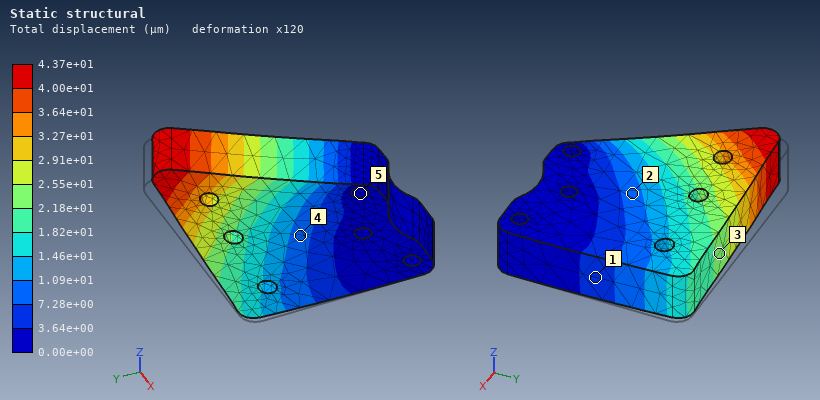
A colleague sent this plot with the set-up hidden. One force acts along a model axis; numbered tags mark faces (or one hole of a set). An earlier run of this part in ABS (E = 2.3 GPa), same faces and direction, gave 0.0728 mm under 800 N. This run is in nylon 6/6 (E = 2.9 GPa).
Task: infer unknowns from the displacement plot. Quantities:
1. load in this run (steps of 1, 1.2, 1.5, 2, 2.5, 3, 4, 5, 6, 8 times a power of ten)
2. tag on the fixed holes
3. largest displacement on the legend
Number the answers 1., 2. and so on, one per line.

1. 600 N
2. 5
3. 4.37e+01 µm
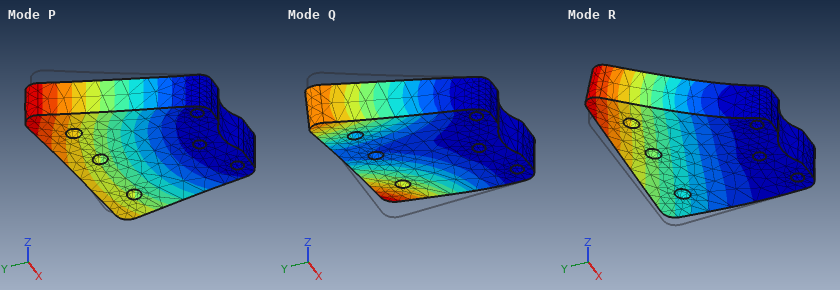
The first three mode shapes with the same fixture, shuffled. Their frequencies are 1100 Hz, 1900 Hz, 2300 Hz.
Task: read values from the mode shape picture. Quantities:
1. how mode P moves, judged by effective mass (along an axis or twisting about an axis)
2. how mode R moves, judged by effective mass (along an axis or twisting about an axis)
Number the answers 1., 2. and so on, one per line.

1. along X
2. along Z
